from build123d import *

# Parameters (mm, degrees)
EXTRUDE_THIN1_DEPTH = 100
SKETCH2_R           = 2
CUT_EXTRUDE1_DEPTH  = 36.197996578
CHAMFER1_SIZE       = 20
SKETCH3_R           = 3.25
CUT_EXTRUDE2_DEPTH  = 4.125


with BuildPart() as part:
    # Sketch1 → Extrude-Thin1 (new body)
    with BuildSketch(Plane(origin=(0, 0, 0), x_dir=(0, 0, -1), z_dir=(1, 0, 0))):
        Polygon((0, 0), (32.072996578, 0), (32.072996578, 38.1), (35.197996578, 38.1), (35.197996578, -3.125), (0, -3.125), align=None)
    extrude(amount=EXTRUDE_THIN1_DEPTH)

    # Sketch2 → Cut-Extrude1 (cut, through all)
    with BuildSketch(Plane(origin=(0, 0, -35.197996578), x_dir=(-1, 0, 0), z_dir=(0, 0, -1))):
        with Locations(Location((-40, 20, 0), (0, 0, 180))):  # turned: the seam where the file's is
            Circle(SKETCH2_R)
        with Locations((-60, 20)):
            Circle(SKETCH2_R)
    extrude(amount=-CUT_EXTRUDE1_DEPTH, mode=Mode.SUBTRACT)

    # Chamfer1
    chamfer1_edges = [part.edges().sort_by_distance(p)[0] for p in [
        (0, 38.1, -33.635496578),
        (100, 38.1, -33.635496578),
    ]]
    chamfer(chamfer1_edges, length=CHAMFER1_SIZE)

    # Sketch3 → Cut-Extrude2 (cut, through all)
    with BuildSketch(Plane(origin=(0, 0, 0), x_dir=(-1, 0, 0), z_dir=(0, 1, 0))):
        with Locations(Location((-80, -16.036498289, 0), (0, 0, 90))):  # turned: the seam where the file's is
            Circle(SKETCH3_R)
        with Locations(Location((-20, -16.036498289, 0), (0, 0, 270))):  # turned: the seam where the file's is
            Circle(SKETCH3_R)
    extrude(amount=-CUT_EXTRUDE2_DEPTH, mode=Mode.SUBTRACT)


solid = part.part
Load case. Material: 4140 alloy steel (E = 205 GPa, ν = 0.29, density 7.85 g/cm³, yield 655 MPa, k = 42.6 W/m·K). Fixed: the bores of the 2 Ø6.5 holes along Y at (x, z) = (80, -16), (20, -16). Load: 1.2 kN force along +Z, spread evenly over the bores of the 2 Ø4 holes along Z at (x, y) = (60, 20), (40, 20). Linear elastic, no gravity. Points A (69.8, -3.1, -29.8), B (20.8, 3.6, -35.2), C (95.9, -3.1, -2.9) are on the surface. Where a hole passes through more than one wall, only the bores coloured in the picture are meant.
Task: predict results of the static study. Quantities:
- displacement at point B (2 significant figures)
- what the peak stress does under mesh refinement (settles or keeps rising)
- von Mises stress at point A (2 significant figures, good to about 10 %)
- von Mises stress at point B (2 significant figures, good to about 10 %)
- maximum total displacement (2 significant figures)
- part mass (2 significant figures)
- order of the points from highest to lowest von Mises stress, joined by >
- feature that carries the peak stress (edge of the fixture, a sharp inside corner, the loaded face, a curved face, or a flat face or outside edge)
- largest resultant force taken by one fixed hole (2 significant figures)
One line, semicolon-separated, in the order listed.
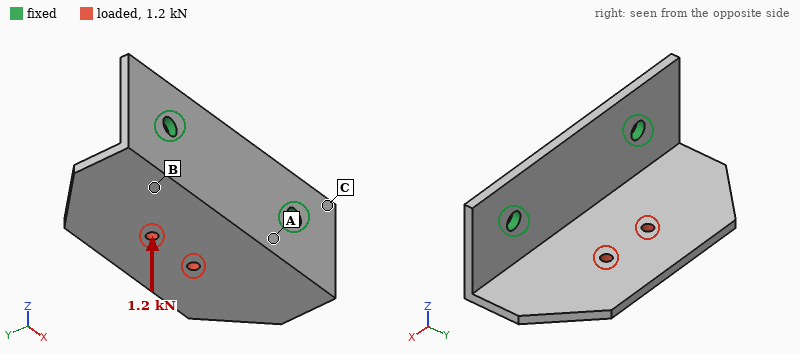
0.11 mm; keeps rising; 160 MPa; 110 MPa; 0.57 mm; 170 g; A > B > C; edge of the fixture; 620 N
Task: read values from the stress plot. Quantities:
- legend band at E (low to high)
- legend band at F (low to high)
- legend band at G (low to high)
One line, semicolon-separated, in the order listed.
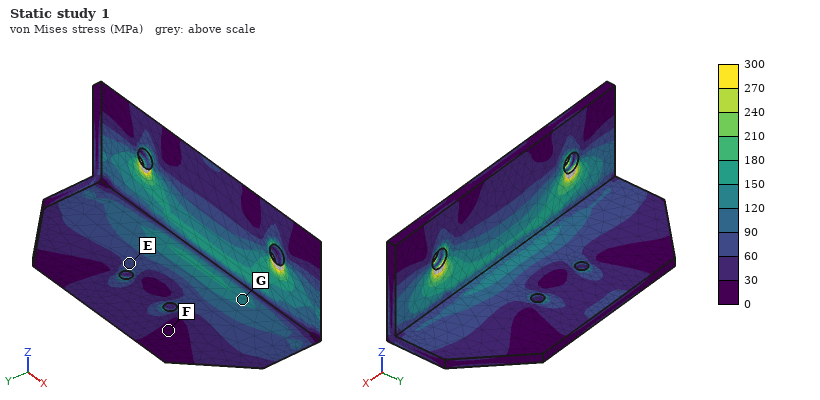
60 to 90 MPa; 0 to 30 MPa; 120 to 150 MPa
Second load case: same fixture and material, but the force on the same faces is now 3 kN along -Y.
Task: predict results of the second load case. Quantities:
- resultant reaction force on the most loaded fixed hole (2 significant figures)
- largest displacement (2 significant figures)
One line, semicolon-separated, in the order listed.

1.5 kN; 0.42 mm
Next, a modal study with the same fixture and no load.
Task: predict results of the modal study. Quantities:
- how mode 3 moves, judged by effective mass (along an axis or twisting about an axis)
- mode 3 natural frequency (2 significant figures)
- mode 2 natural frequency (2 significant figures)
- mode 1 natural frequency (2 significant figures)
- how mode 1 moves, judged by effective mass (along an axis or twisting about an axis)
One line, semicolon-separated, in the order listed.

along Y; 3300 Hz; 2000 Hz; 1100 Hz; along Z
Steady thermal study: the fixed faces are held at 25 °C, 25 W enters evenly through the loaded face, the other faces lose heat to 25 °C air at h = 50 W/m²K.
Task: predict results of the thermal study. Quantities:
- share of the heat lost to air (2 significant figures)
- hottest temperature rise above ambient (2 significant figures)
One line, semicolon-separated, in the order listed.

65 %; 75 K
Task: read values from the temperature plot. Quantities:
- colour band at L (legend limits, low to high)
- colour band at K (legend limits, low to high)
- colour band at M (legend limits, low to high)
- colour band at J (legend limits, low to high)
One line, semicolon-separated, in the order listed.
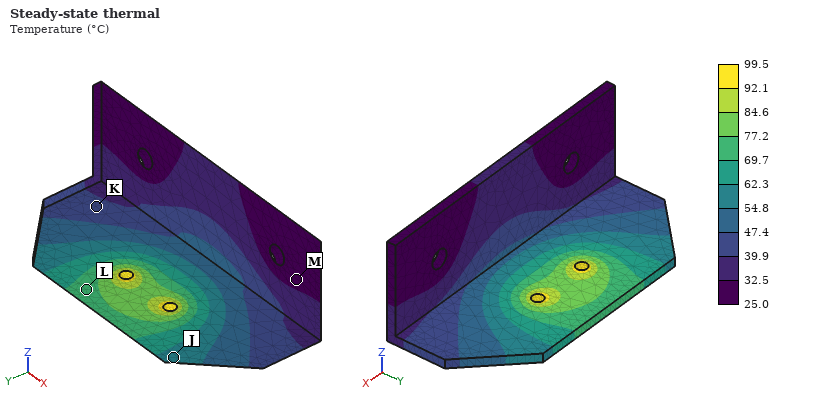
69.7 to 77.2 °C; 39.9 to 47.4 °C; 25.0 to 32.5 °C; 54.8 to 62.3 °C
